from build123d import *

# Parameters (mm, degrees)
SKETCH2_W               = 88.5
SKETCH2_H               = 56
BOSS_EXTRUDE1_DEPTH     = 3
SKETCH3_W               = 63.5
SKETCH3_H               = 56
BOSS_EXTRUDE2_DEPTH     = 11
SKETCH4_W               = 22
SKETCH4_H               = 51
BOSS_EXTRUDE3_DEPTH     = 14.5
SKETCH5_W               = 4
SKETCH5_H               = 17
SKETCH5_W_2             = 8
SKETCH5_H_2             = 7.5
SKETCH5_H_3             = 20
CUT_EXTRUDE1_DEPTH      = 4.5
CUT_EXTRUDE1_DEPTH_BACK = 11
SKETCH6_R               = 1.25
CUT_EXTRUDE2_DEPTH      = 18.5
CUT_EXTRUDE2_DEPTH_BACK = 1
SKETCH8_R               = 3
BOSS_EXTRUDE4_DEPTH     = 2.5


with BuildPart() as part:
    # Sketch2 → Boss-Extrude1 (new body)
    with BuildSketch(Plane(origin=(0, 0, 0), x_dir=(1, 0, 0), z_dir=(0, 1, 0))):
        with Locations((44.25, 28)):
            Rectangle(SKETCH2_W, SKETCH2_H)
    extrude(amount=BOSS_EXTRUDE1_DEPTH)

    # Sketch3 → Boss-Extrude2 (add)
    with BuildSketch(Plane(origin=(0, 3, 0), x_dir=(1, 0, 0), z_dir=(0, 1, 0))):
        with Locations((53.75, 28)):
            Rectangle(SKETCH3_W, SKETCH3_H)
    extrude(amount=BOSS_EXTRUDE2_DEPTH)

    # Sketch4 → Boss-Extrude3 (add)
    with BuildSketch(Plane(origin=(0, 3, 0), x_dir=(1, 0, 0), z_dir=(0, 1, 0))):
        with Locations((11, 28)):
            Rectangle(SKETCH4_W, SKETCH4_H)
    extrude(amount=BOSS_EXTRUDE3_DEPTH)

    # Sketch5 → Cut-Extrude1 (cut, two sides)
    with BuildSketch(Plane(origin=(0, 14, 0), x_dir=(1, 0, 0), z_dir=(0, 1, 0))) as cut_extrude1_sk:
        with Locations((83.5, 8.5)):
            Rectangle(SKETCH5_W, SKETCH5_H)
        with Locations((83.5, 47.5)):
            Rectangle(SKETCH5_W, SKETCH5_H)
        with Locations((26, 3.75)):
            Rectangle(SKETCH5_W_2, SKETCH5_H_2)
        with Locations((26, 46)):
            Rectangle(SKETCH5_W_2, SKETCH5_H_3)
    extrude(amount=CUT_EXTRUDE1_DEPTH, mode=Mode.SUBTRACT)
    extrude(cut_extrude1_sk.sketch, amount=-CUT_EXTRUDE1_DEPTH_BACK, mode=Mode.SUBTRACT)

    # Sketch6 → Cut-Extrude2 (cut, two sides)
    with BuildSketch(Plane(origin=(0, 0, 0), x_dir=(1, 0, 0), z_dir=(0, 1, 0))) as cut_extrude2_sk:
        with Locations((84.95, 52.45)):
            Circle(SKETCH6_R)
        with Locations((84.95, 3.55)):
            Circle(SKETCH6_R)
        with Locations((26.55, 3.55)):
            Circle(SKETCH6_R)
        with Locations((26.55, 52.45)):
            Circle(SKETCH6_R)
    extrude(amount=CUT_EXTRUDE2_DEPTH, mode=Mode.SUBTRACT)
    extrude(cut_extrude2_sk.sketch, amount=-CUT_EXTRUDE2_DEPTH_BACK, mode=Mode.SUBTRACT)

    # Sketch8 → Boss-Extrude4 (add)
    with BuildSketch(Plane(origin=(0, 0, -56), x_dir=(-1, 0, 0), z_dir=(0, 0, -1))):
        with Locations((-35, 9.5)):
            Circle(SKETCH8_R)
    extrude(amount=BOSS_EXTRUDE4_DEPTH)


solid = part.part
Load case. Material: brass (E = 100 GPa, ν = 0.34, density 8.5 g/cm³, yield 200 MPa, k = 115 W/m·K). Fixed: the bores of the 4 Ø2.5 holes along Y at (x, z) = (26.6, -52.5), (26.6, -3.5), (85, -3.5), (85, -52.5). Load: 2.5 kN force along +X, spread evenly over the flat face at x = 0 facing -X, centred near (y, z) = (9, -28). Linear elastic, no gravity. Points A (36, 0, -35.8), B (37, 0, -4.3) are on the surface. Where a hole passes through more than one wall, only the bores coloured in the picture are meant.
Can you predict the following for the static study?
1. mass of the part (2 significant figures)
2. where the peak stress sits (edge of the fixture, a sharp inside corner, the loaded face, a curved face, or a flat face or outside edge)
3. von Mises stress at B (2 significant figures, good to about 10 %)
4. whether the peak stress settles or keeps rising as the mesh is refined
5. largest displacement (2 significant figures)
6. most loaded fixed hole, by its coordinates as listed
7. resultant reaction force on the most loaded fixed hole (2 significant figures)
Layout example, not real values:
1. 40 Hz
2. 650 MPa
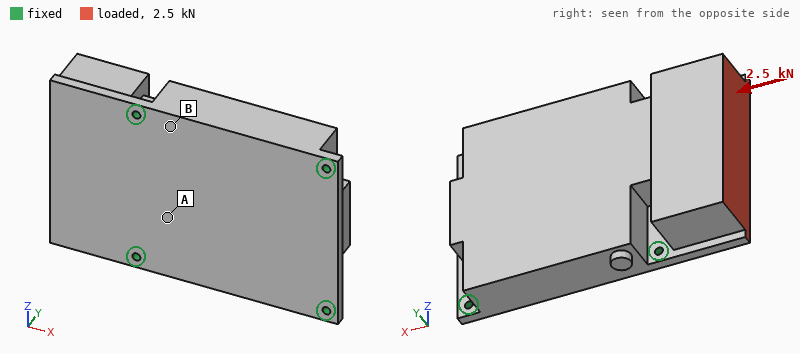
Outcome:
1. 560 g
2. edge of the fixture
3. 8.1 MPa
4. keeps rising
5. 14 µm
6. (26.6, -52.5)
7. 850 N
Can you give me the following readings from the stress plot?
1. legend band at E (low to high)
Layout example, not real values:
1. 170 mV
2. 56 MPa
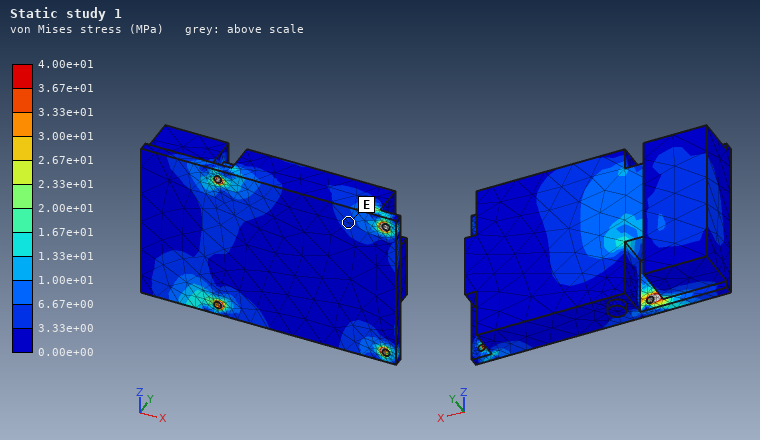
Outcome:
1. 3.33e+00 to 6.67e+00 MPa
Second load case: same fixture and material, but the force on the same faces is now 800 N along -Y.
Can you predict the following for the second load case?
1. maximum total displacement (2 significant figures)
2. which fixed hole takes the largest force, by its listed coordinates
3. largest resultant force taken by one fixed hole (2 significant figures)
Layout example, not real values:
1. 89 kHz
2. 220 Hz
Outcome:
1. 26 µm
2. (26.6, -3.5)
3. 780 N
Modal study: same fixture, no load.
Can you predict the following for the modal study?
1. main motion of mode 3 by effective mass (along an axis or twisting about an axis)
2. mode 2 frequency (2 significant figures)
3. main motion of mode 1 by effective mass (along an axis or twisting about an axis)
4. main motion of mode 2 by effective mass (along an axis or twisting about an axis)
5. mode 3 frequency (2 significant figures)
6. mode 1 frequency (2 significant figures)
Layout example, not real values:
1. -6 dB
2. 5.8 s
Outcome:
1. along Z
2. 4500 Hz
3. along Y
4. along Y
5. 6000 Hz
6. 3100 Hz
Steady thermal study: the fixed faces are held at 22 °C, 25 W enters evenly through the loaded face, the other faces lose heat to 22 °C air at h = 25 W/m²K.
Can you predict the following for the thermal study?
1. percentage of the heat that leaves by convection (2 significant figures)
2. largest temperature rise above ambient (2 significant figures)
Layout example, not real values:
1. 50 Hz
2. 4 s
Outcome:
1. 11 %
2. 17 K
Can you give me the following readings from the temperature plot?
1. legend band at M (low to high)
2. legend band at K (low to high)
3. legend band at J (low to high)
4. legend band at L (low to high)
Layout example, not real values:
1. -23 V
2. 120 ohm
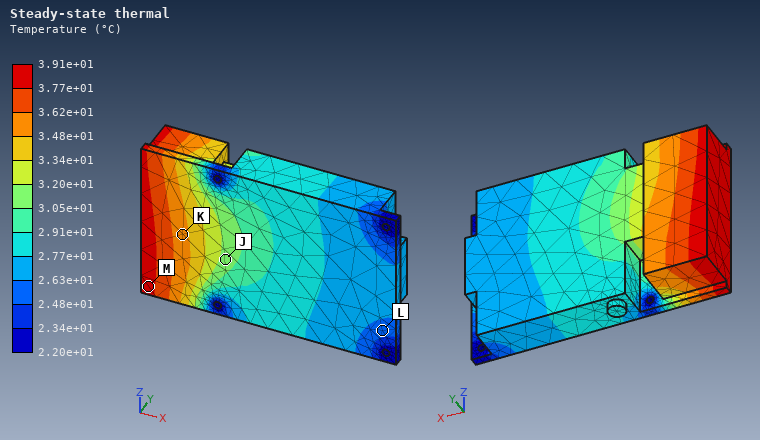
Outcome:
1. 3.77e+01 to 3.91e+01 °C
2. 3.48e+01 to 3.62e+01 °C
3. 3.05e+01 to 3.20e+01 °C
4. 2.48e+01 to 2.63e+01 °C
